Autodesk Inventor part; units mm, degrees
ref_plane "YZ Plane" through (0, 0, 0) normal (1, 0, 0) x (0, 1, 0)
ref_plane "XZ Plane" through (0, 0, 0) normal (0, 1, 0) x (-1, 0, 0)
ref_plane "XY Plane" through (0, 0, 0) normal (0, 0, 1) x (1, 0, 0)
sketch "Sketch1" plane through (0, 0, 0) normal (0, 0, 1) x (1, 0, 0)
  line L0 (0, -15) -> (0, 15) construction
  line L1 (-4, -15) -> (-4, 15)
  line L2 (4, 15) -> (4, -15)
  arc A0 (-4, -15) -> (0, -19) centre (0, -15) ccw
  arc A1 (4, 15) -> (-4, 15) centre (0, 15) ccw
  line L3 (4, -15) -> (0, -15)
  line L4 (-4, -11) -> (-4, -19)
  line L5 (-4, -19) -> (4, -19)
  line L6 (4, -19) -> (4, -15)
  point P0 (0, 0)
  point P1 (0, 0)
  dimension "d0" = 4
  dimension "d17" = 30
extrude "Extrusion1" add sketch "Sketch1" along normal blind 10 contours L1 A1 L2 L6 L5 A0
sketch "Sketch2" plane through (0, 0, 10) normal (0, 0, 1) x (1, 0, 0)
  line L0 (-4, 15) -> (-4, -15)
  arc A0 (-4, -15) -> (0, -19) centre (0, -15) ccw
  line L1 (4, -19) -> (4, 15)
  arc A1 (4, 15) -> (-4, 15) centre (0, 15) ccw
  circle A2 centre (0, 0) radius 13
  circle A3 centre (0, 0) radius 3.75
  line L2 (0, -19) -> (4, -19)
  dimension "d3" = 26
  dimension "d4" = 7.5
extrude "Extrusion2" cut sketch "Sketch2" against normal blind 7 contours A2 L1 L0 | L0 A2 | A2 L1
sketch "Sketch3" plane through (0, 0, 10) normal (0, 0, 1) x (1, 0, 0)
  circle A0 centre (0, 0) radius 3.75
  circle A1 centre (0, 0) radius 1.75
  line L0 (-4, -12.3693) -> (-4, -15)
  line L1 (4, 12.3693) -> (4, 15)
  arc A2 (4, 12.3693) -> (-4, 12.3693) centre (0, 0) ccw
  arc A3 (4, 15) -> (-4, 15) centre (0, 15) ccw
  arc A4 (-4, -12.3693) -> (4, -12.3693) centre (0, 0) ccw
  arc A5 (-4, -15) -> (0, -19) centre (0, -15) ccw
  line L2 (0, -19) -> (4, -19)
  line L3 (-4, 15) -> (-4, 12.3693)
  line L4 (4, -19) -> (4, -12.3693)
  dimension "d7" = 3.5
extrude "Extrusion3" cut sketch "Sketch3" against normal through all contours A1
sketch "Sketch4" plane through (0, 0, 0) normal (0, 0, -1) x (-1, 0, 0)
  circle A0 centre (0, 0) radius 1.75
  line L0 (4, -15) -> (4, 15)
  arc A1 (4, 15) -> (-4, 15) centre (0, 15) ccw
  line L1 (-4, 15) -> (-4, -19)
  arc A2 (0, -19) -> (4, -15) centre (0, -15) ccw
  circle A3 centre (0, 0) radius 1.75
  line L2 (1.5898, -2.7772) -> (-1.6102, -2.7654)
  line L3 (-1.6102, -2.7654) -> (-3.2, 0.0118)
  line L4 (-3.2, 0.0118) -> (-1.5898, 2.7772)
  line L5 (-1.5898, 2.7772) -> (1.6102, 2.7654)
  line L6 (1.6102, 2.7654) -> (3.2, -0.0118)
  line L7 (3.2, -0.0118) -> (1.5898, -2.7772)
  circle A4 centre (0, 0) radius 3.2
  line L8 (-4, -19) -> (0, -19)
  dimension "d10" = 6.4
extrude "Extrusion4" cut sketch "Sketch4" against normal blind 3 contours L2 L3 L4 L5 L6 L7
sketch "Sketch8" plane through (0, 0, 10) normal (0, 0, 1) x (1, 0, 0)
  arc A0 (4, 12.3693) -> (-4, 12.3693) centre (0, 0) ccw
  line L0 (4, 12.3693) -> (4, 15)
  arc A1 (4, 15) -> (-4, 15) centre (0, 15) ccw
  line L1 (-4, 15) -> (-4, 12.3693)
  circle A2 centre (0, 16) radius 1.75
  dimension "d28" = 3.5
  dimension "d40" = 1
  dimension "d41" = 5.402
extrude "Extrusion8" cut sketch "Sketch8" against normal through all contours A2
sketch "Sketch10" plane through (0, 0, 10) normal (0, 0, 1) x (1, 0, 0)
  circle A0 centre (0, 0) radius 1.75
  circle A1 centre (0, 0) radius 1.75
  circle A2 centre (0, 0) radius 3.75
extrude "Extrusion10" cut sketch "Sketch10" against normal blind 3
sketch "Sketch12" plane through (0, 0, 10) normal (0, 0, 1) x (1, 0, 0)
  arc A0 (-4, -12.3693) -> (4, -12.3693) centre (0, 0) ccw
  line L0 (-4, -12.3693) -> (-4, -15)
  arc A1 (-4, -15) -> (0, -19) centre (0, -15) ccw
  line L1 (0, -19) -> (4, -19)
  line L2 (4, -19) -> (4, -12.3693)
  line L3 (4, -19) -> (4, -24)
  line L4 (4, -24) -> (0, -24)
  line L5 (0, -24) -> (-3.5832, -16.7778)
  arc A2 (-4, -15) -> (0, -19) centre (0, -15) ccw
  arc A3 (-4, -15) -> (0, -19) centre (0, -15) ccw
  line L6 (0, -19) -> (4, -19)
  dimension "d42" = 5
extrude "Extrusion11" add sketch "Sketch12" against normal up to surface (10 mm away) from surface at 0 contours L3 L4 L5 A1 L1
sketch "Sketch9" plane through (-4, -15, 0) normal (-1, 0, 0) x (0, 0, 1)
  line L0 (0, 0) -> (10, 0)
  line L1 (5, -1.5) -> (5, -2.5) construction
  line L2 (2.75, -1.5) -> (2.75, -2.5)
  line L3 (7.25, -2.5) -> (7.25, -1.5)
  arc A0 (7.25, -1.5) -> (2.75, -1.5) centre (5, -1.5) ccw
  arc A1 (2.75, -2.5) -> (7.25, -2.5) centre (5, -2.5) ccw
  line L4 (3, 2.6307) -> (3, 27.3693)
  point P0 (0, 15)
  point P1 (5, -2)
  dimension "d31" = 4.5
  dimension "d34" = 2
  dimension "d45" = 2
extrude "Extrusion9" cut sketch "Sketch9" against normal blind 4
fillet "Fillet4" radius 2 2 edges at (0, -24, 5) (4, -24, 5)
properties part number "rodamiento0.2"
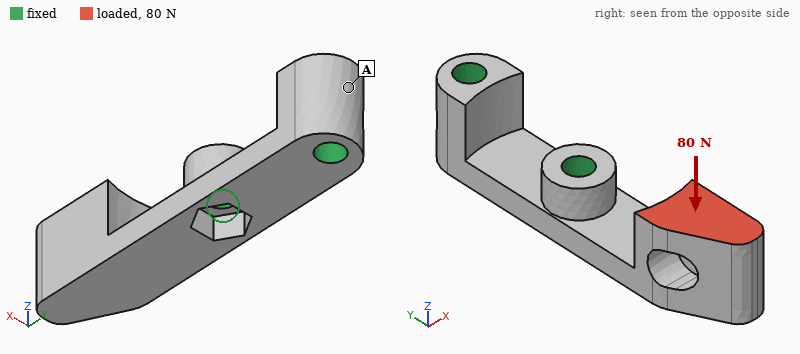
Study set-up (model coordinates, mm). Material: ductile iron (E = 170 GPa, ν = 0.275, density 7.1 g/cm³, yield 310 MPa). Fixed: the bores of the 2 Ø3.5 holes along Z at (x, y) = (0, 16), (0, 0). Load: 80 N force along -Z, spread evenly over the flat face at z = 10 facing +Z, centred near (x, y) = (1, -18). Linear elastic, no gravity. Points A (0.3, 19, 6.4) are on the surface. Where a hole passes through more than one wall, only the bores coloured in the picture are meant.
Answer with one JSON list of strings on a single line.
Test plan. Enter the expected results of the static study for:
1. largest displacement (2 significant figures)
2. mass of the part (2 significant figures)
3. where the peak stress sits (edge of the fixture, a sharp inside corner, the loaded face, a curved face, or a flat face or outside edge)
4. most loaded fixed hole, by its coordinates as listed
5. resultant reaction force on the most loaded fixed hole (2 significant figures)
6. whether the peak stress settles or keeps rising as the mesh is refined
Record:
["82 µm", "12 g", "a sharp inside corner", "(0, 0)", "150 N", "keeps rising"]
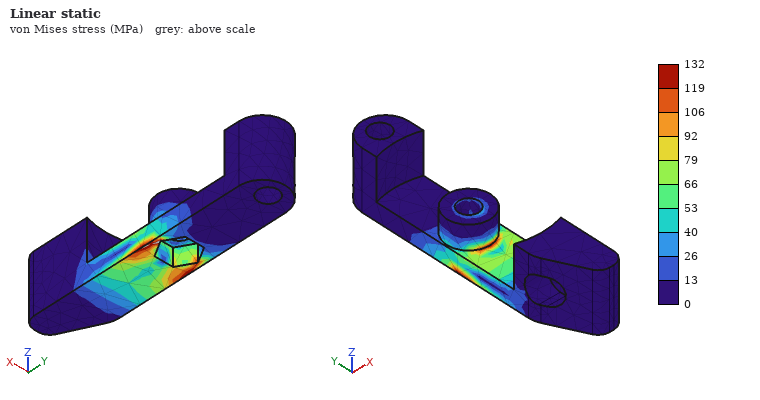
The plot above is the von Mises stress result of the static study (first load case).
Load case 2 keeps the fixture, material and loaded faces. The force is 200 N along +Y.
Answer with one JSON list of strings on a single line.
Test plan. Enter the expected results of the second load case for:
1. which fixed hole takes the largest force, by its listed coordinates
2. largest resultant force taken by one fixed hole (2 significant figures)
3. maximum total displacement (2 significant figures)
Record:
["(0, 0)", "300 N", "0.15 mm"]
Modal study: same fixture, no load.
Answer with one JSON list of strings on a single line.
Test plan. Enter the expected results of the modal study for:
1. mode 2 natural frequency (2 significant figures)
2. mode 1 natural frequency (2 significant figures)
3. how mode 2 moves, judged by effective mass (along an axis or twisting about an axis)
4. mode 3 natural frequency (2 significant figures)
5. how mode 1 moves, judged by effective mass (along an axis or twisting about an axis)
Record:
["5000 Hz", "2700 Hz", "along X", "12 kHz", "along Z"]
